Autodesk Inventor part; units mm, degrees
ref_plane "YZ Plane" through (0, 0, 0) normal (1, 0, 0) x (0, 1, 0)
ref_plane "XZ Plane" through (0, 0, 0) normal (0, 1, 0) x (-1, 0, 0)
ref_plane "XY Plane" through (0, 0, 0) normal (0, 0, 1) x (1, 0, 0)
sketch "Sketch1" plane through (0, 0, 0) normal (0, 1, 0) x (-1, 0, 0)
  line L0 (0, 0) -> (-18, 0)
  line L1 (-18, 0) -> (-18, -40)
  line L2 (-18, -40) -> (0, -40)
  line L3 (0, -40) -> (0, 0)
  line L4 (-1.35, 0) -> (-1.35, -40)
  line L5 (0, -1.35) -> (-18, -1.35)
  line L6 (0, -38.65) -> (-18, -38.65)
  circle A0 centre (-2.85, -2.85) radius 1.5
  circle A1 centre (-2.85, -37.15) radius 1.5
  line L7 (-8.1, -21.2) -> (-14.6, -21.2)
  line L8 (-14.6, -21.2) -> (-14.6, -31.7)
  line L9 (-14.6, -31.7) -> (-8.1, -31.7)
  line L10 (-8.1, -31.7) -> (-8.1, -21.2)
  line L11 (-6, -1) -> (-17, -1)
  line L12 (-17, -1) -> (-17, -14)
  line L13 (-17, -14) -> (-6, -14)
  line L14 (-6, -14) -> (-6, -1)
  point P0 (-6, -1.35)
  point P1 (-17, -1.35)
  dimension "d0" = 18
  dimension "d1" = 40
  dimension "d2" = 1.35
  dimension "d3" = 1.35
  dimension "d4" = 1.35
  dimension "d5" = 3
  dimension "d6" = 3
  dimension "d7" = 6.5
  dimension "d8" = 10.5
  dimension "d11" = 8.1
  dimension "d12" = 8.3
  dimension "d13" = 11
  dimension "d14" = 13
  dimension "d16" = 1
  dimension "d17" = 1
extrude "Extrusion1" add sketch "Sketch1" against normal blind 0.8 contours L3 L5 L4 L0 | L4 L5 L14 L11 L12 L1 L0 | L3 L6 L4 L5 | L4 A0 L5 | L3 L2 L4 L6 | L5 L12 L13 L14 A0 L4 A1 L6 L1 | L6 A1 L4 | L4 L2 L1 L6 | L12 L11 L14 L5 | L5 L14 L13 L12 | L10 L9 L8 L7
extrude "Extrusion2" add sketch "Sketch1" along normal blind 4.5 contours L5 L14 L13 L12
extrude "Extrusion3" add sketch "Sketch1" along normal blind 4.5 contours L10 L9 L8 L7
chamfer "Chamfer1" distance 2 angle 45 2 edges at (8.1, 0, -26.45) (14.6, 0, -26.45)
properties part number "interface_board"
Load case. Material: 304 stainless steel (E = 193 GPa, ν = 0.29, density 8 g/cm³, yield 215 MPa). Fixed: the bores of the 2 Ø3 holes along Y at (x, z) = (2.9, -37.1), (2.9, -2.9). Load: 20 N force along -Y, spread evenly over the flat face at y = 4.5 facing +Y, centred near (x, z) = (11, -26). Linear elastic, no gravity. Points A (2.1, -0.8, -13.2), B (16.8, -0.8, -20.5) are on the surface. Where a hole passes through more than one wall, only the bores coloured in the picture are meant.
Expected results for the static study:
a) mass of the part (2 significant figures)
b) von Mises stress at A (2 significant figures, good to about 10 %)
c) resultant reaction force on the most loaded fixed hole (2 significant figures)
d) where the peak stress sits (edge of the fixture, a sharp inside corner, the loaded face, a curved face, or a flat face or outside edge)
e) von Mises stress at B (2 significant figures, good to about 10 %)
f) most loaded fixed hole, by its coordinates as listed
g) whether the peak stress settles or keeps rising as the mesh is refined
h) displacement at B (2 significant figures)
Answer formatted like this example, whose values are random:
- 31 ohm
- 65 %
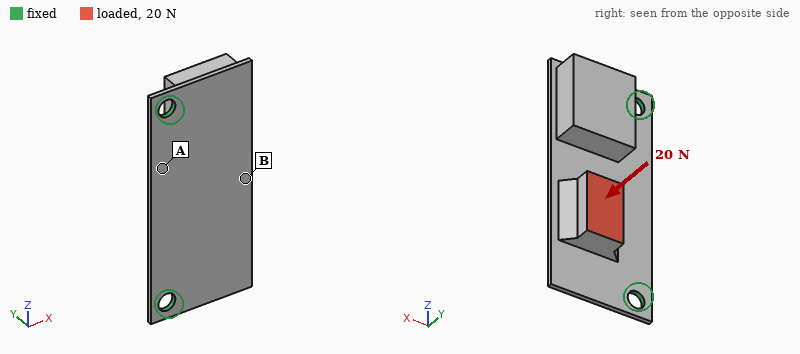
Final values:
- 12 g
- 13 MPa
- 13 N
- edge of the fixture
- 34 MPa
- (2.9, -37.1)
- keeps rising
- 47 µm
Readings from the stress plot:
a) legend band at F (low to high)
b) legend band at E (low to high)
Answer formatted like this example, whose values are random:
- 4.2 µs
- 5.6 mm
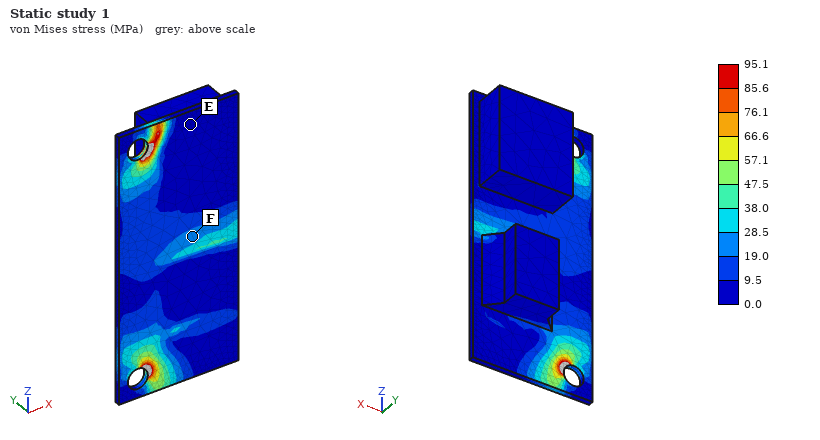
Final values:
- 19.0 to 28.5 MPa
- 0.0 to 9.5 MPa
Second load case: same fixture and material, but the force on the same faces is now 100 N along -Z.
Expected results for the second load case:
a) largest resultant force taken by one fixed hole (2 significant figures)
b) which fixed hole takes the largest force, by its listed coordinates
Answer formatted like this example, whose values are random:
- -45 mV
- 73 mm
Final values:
- 64 N
- (2.9, -37.1)
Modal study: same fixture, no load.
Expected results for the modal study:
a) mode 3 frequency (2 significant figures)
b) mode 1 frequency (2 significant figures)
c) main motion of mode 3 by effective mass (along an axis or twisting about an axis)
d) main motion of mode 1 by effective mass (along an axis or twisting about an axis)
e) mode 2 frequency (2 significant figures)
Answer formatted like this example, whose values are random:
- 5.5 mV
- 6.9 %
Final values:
- 4200 Hz
- 1300 Hz
- twisting about X
- along Y
- 3600 Hz
